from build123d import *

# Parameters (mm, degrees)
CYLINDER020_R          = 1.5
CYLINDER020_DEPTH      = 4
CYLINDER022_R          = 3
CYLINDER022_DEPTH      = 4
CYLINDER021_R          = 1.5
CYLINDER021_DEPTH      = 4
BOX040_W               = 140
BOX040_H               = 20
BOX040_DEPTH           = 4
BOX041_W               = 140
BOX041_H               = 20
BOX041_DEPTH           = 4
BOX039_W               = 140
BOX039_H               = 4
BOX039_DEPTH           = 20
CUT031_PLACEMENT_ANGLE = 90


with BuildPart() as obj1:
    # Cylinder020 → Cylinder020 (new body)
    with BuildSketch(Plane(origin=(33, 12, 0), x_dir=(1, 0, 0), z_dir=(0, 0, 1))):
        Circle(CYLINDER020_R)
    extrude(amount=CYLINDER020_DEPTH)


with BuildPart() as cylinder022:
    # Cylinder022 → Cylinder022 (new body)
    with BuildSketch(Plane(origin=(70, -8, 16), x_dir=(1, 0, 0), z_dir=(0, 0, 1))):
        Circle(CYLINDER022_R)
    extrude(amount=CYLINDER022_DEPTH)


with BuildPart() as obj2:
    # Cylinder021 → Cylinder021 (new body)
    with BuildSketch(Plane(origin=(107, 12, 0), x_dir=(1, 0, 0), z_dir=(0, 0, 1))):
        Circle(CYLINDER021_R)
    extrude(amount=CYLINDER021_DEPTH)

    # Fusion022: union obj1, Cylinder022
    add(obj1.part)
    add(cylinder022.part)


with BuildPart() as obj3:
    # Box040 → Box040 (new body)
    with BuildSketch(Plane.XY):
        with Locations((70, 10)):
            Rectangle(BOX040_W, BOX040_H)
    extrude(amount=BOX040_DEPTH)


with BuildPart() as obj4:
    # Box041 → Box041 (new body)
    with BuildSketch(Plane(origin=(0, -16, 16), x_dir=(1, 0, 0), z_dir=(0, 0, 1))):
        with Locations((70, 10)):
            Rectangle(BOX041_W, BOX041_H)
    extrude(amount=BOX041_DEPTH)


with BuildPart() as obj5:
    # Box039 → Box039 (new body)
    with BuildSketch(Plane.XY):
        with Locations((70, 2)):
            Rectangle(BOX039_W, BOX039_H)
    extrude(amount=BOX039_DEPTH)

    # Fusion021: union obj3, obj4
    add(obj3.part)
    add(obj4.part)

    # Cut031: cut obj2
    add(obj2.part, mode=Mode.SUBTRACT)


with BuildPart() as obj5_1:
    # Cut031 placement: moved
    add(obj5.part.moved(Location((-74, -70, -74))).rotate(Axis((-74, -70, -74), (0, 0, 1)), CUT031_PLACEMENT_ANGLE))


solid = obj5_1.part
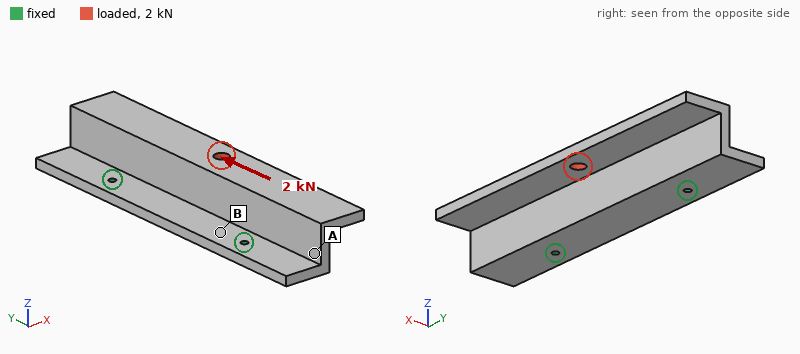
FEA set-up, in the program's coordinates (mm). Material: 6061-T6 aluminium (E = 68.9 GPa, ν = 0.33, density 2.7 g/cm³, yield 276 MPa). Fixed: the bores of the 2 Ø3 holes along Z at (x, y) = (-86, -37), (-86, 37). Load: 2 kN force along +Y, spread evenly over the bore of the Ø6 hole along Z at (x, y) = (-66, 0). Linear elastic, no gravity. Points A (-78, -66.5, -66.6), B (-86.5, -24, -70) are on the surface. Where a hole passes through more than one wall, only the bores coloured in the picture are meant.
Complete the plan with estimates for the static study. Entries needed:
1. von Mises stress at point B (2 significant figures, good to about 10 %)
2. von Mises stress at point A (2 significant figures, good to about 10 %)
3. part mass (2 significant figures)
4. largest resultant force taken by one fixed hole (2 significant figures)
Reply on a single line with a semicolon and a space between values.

15 MPa; 6.2 MPa; 78 g; 1.2 kN
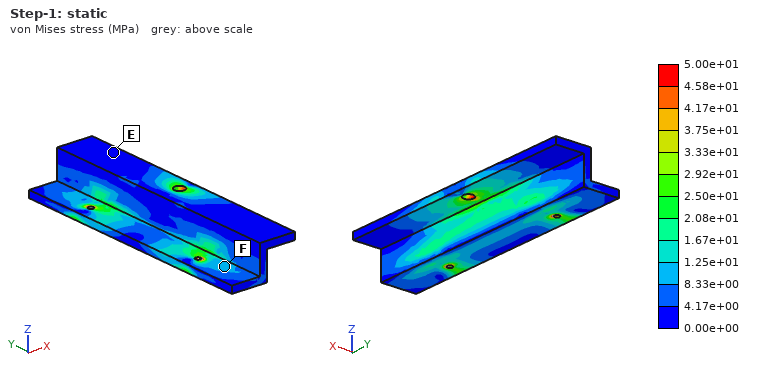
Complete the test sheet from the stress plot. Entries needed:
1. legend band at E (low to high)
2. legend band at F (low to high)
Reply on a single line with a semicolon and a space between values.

0.00e+00 to 4.17e+00 MPa; 8.33e+00 to 1.25e+01 MPa
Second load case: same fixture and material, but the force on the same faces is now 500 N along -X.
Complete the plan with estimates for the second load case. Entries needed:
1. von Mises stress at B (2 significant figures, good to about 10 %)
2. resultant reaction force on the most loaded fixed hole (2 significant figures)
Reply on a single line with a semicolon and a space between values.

25 MPa; 250 N
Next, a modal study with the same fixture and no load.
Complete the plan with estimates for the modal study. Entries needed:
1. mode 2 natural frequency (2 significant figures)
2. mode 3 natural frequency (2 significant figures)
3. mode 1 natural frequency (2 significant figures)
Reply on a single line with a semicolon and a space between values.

2200 Hz; 3700 Hz; 1600 Hz
